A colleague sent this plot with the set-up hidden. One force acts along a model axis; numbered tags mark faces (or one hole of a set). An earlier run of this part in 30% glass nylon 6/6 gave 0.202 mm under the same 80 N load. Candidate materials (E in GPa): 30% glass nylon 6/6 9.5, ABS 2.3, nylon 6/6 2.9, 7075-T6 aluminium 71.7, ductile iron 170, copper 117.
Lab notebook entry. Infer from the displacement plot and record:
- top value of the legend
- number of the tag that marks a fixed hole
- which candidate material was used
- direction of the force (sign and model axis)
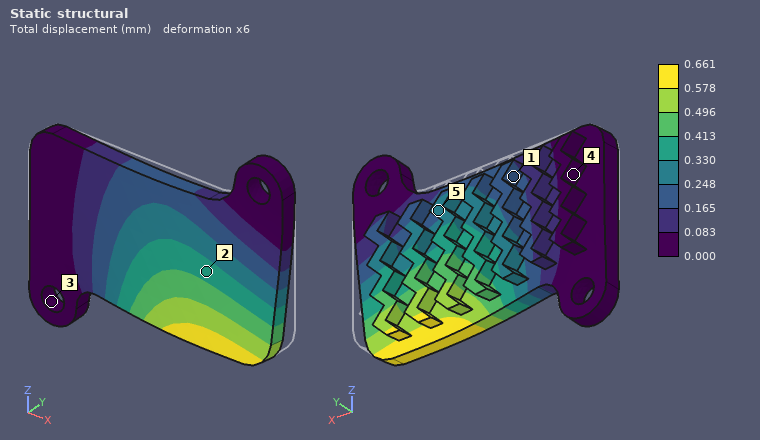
0.661 mm
3
nylon 6/6
-Y
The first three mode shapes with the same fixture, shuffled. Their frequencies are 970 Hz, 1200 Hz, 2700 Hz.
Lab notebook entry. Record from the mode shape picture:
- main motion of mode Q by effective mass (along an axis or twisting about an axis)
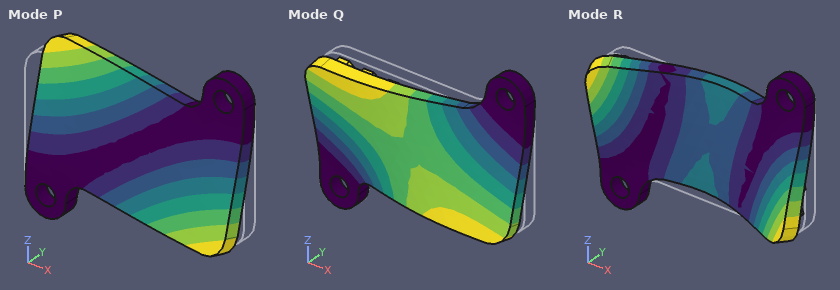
along Y
